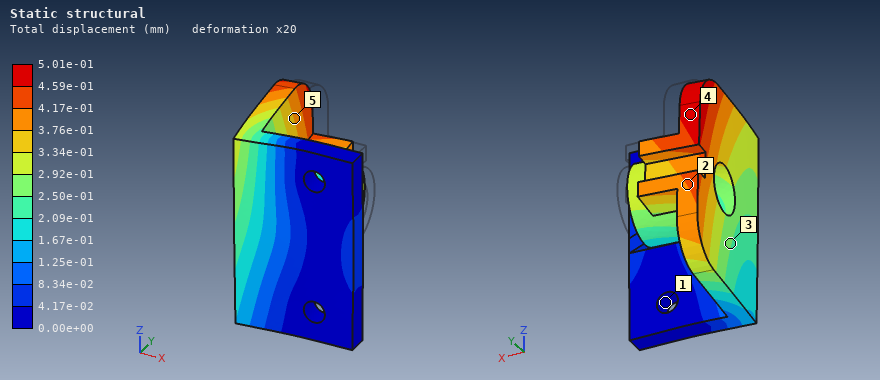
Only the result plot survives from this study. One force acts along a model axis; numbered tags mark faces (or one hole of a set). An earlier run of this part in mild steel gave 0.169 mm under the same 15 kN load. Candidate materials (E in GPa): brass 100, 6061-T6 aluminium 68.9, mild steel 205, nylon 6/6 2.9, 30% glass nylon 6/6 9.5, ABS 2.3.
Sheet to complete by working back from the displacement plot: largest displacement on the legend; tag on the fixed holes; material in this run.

5.01e-01 mm
1
6061-T6 aluminium
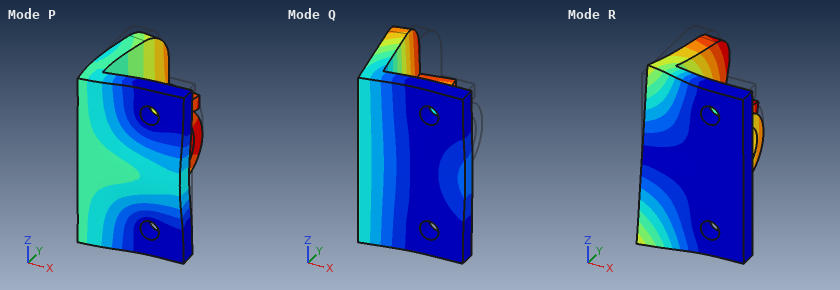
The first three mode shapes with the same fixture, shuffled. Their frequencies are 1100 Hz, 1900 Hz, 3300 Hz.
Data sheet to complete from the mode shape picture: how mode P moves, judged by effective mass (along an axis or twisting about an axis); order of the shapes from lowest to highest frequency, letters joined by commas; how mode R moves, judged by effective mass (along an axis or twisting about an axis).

along Y
Q, R, P
along Z
